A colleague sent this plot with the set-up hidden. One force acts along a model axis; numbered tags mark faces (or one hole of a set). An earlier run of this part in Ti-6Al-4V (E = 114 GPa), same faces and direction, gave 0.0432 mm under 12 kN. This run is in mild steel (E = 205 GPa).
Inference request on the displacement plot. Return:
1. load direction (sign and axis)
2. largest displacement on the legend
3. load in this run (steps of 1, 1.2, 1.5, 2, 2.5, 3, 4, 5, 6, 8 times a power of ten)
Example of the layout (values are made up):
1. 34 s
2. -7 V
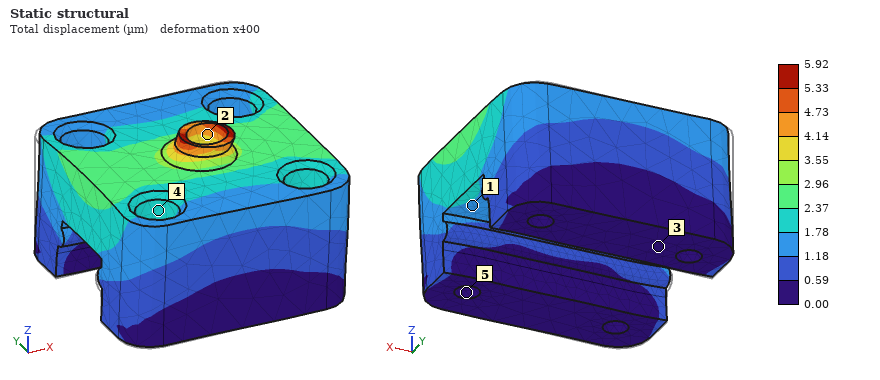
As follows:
1. +X
2. 5.92 µm
3. 3 kN
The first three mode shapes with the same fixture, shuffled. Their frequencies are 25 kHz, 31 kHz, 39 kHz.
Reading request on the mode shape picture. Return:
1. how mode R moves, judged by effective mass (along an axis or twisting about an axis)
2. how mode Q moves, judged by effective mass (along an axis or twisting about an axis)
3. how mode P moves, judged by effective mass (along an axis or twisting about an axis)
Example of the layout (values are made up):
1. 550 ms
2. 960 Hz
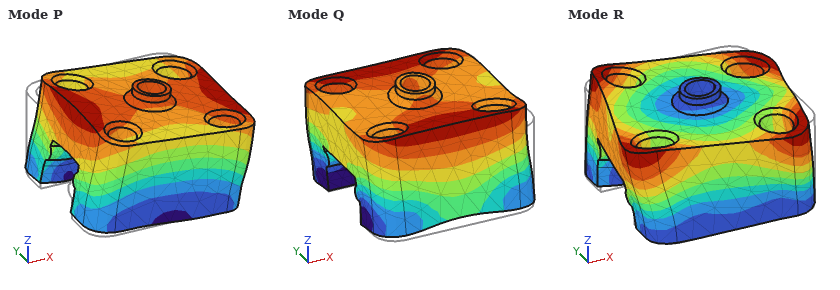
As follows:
1. twisting about Z
2. along Y
3. along X
